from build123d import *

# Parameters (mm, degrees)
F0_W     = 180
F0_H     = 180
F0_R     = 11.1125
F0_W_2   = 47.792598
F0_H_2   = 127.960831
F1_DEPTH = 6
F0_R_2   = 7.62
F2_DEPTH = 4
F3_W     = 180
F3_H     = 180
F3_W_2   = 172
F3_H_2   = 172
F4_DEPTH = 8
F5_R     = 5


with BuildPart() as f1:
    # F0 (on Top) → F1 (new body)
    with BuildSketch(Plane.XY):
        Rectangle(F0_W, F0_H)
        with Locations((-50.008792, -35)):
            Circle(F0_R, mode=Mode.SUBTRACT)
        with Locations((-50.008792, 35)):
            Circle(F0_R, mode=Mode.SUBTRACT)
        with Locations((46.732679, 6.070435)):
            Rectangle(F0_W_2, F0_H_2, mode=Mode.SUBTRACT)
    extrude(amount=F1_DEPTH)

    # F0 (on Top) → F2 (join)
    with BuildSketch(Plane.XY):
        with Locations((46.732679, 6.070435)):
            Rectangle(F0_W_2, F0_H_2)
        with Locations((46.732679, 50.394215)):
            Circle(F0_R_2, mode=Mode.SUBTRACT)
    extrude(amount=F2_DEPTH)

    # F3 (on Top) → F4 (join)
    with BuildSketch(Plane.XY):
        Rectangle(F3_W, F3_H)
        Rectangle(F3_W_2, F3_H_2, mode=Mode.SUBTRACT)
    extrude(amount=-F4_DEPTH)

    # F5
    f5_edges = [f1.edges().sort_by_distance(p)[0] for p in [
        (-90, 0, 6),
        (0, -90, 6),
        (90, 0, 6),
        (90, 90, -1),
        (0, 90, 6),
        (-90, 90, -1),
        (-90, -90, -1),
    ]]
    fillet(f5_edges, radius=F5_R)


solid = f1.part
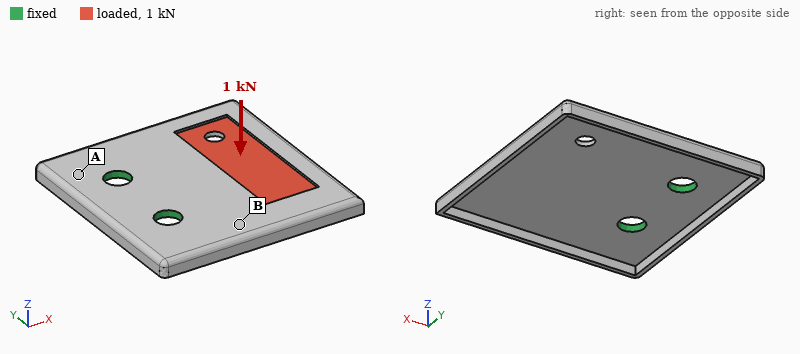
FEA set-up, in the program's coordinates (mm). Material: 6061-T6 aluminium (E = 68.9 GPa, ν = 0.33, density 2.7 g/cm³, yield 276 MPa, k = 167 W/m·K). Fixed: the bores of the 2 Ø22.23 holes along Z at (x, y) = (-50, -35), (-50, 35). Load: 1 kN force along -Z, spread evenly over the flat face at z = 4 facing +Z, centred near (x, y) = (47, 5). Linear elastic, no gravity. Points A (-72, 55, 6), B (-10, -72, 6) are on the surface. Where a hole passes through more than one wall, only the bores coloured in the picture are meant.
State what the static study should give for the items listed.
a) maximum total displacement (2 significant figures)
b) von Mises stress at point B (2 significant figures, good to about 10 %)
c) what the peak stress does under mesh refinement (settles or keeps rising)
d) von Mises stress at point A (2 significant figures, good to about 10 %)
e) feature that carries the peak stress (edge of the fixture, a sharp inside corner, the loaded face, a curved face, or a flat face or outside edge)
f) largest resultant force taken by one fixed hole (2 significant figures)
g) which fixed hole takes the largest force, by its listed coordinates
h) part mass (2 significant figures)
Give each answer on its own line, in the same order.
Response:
1.5 mm
31 MPa
keeps rising
13 MPa
edge of the fixture
550 N
(-50, 35)
530 g
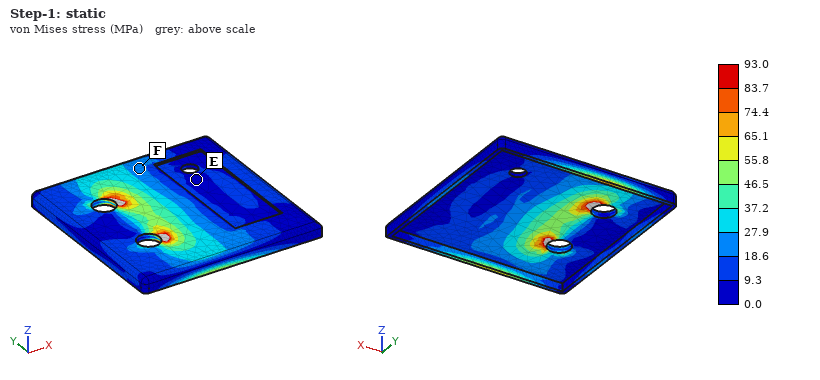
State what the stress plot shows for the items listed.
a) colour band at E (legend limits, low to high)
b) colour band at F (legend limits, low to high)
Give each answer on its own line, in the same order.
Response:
0.0 to 9.3 MPa
18.6 to 27.9 MPa
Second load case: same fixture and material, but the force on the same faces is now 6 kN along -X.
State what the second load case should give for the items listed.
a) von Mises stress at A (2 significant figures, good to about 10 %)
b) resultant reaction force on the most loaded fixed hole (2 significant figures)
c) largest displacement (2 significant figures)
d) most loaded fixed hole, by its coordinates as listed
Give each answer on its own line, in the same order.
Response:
3.3 MPa
3.4 kN
0.21 mm
(-50, 35)
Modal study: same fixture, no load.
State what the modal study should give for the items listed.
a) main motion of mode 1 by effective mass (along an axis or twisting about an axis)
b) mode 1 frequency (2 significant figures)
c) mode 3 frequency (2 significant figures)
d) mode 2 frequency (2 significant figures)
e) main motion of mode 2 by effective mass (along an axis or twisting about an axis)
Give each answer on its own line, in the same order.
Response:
along Z
310 Hz
1300 Hz
460 Hz
twisting about X
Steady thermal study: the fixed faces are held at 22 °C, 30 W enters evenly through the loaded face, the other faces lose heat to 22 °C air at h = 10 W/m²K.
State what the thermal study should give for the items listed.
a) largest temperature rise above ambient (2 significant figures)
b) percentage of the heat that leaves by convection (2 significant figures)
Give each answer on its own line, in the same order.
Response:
16 K
17 %
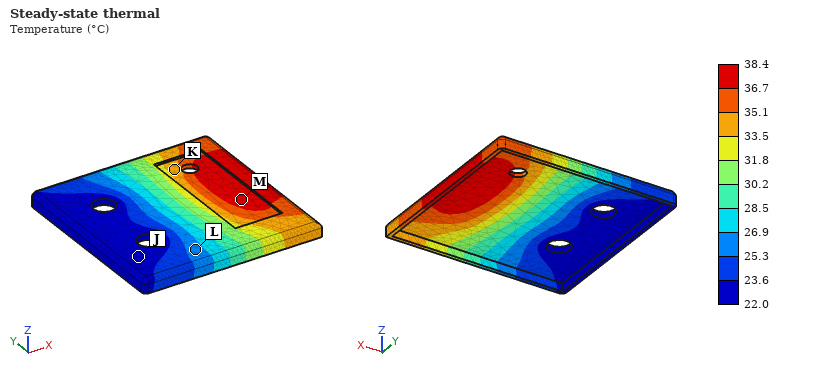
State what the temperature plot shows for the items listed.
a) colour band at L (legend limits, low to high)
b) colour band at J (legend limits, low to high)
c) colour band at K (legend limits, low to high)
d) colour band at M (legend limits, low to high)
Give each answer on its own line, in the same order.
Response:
25.3 to 26.9 °C
22.0 to 23.6 °C
33.5 to 35.1 °C
36.7 to 38.4 °C
